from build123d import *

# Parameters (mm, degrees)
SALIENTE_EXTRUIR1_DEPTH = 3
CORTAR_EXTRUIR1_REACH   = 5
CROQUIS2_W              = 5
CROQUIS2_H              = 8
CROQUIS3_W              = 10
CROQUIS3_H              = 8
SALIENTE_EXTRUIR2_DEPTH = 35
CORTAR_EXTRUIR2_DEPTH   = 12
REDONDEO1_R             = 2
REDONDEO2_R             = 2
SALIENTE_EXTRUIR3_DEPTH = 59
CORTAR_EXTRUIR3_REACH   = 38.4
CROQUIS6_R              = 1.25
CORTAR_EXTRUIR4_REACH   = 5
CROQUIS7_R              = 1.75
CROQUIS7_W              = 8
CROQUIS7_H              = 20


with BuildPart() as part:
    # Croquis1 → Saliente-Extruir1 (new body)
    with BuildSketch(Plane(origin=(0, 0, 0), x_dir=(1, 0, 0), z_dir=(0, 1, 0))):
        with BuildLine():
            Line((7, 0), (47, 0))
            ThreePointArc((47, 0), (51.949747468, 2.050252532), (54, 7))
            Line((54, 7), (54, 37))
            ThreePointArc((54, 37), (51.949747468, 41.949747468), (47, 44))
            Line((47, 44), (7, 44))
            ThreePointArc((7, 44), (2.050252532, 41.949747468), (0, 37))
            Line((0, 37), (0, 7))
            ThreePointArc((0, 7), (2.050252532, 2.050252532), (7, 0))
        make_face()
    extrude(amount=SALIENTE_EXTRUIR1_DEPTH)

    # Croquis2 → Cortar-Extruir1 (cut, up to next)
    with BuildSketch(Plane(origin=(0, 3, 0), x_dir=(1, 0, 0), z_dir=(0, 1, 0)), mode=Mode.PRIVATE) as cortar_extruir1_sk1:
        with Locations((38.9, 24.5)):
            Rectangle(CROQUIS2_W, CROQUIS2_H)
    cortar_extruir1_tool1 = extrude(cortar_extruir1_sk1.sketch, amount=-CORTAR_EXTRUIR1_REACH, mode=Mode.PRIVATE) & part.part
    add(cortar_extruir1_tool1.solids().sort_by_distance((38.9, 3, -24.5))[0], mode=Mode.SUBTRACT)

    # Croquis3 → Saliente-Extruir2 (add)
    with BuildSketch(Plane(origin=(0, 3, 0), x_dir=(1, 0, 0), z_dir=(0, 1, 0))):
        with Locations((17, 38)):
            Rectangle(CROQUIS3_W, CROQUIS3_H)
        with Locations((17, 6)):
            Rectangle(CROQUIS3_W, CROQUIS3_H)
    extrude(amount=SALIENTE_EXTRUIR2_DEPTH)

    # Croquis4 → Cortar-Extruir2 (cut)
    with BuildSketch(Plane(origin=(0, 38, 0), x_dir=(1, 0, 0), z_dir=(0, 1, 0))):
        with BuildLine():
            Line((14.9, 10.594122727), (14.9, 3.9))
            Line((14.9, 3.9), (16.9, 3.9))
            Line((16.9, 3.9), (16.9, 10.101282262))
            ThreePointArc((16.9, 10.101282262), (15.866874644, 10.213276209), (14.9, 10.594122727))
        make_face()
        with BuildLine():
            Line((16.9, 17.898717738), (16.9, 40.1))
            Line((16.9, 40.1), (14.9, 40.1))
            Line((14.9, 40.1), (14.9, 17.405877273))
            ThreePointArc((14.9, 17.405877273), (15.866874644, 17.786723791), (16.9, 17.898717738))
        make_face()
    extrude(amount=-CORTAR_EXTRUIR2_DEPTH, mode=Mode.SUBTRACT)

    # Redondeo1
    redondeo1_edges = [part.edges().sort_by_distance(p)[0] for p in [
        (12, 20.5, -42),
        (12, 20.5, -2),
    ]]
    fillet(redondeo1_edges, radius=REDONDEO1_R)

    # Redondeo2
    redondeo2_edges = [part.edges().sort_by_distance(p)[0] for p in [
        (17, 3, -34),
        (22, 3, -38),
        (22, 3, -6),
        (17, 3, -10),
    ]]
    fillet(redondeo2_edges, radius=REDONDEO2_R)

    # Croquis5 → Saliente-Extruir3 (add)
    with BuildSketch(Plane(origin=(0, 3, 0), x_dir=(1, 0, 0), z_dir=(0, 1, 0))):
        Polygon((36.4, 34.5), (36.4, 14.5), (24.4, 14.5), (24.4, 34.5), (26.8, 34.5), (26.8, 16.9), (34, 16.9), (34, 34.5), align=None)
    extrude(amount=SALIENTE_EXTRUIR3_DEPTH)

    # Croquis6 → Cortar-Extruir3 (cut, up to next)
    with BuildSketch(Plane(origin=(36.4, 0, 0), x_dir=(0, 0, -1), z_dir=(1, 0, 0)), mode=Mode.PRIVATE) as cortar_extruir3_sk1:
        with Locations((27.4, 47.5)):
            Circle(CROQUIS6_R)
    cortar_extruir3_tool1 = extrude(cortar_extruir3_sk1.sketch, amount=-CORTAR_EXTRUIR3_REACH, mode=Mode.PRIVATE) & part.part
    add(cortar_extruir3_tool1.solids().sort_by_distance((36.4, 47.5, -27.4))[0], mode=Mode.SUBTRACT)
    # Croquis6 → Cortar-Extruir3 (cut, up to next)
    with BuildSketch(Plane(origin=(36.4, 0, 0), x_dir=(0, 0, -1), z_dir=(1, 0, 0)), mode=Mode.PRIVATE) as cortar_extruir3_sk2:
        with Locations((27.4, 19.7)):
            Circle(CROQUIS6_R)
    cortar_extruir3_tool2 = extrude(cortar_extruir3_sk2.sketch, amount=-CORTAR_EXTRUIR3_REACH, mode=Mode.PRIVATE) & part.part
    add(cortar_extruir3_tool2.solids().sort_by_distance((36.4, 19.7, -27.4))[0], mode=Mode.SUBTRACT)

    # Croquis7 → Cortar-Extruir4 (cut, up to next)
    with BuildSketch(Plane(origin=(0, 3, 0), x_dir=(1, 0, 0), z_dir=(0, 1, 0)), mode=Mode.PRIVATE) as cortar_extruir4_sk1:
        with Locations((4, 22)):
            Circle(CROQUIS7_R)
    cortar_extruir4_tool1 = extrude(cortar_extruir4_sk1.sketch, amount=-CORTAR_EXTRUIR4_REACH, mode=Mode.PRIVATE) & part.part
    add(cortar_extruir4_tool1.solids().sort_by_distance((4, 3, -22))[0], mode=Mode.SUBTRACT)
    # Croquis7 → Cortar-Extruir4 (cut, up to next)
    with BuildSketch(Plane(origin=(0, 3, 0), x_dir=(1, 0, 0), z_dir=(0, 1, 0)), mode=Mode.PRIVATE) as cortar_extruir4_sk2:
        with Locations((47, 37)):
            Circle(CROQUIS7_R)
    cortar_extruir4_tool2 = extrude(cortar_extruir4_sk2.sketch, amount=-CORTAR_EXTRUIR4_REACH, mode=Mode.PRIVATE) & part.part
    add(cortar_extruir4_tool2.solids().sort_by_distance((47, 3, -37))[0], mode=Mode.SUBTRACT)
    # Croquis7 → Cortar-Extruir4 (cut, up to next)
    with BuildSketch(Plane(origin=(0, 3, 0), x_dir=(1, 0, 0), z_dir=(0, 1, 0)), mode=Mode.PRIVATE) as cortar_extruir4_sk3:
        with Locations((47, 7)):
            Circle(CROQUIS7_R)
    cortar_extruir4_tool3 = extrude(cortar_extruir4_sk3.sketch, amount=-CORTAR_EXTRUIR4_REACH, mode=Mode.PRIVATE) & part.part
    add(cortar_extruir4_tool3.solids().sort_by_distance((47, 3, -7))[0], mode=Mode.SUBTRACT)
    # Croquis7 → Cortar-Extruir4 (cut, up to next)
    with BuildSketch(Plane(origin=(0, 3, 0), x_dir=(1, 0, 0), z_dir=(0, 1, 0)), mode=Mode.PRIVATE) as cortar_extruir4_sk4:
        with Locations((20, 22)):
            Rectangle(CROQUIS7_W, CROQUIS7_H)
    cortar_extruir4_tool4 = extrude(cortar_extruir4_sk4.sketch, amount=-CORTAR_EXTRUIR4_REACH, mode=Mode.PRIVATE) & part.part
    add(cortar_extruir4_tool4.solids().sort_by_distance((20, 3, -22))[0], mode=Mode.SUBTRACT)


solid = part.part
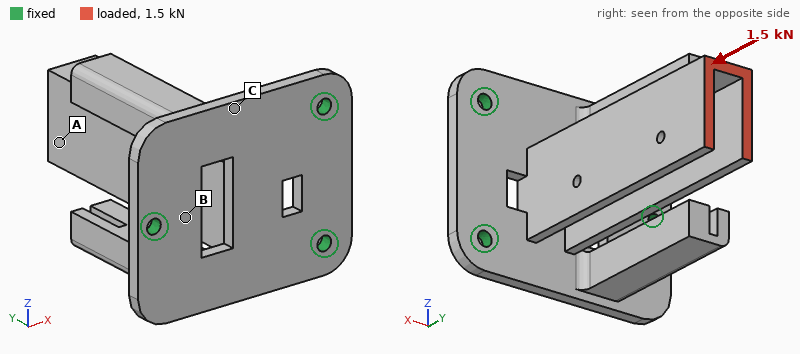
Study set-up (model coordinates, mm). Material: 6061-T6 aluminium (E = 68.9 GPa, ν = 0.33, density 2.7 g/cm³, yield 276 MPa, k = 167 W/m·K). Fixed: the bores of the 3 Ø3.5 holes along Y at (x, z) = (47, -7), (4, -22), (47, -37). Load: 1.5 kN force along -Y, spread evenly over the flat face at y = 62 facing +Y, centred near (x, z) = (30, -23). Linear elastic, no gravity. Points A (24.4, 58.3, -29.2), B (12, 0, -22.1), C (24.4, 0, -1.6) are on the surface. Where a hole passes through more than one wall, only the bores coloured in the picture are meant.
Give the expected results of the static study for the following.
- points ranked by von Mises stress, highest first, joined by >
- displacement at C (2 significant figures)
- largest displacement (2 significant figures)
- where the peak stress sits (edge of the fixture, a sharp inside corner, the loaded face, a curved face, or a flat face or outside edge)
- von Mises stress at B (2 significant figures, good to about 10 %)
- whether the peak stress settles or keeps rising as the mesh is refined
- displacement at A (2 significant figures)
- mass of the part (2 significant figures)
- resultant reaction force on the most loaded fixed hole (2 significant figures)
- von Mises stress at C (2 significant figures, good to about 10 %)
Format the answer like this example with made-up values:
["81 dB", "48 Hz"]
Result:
["C > B > A", "0.091 mm", "0.35 mm", "edge of the fixture", "58 MPa", "keeps rising", "0.33 mm", "49 g", "550 N", "100 MPa"]
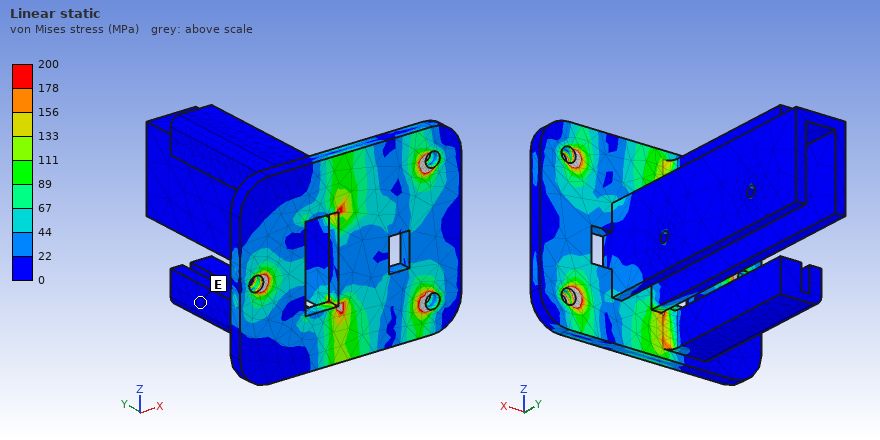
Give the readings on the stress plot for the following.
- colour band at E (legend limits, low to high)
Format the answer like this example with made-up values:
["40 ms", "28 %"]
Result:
["0 to 22 MPa"]
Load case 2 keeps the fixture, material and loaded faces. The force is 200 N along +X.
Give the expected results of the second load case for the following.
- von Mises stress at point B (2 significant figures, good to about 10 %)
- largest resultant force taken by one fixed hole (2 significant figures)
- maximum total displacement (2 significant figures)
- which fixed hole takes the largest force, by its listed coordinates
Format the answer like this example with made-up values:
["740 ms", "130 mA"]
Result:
["37 MPa", "330 N", "1.0 mm", "(4, -22)"]
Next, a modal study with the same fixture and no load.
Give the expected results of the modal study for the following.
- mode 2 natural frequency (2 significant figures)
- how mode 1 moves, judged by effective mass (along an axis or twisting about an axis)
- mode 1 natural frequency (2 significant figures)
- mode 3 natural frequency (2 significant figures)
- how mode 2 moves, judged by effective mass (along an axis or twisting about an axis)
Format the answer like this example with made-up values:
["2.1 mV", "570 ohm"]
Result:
["1400 Hz", "along X", "1000 Hz", "1700 Hz", "along Z"]
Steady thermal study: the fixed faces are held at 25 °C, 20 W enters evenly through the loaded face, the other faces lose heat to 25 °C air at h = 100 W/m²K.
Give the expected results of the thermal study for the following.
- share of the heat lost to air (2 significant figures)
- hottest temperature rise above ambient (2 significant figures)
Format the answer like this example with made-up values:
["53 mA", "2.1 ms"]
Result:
["70 %", "43 K"]
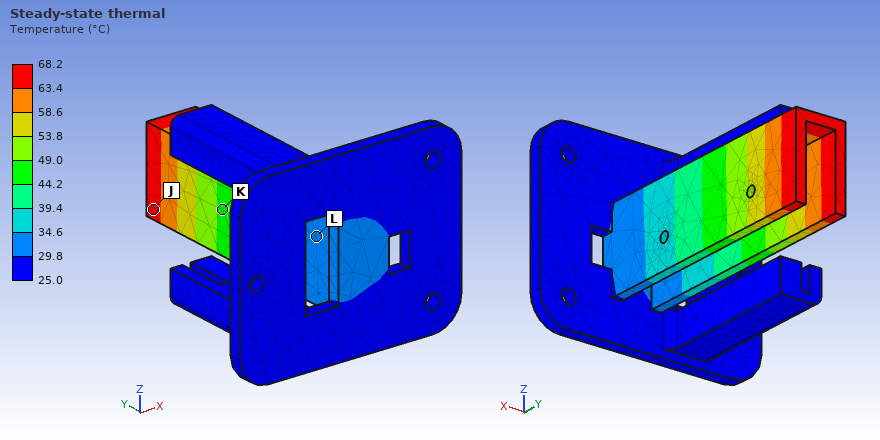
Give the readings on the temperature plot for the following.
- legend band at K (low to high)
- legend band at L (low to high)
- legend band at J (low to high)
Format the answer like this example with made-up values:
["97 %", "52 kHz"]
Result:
["44.2 to 49.0 °C", "29.8 to 34.6 °C", "63.4 to 68.2 °C"]
